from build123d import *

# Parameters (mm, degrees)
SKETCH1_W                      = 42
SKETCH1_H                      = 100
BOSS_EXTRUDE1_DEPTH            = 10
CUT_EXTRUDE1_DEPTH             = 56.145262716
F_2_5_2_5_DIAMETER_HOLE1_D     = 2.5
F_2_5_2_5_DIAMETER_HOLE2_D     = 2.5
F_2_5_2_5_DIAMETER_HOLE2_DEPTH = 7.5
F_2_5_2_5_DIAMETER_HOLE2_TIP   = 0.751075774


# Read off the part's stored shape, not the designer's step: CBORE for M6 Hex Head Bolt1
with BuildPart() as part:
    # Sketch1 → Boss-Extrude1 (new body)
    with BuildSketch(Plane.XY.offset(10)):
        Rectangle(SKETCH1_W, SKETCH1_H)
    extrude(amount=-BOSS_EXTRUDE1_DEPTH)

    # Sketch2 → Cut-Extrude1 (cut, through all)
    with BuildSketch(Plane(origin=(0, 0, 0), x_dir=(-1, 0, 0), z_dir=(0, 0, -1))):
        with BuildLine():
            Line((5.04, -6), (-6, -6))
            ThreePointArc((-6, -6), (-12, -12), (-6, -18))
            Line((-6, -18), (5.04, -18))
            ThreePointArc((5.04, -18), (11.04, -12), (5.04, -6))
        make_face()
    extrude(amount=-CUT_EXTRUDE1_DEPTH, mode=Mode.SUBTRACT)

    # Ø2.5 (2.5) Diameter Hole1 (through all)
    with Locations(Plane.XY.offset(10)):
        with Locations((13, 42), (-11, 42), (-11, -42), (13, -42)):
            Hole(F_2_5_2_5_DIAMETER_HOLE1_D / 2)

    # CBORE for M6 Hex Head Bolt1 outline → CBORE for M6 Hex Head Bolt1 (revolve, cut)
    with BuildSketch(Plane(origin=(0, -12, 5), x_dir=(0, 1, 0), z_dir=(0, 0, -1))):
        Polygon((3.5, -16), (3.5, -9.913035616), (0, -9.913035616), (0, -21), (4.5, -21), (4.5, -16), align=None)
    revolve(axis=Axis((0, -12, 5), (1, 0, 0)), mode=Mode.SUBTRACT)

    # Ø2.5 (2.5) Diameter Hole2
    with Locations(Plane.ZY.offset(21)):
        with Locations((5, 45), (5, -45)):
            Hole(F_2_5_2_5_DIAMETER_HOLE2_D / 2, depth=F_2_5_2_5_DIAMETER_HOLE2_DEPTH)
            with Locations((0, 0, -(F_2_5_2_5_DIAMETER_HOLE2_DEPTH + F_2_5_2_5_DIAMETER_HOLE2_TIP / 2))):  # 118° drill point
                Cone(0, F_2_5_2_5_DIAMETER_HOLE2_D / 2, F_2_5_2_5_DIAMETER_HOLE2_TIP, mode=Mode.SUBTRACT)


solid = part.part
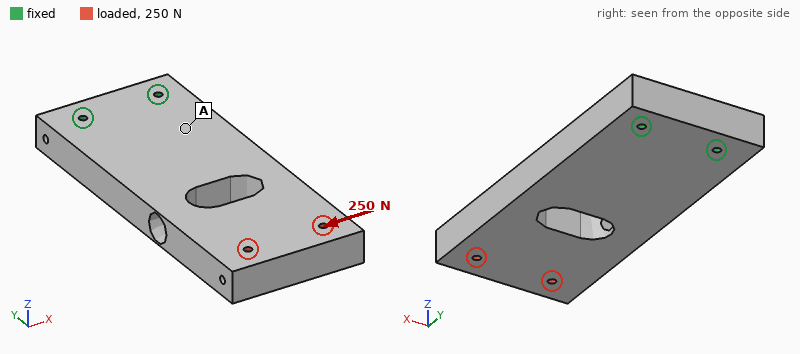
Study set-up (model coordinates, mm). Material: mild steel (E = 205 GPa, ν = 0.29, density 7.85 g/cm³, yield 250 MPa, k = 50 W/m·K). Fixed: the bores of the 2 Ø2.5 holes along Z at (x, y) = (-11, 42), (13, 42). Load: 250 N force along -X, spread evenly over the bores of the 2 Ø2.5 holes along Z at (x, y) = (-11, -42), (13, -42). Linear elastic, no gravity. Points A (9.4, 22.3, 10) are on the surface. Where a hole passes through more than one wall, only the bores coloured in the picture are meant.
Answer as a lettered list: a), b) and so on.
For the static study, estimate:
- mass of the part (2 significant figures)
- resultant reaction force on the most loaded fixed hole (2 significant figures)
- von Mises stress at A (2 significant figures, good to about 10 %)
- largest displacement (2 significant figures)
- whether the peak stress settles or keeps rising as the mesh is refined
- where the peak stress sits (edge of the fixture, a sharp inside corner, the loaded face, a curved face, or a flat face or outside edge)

a) 300 g
b) 850 N
c) 2.9 MPa
d) 8.2 µm
e) keeps rising
f) edge of the fixture
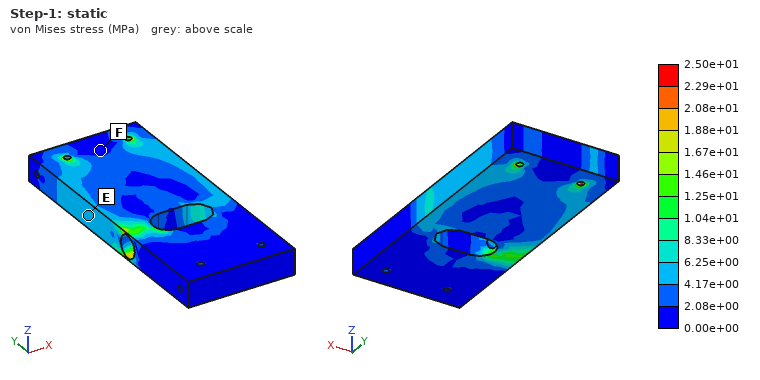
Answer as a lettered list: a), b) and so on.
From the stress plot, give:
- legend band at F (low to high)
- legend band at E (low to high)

a) 0.00e+00 to 2.08e+00 MPa
b) 4.17e+00 to 6.25e+00 MPa
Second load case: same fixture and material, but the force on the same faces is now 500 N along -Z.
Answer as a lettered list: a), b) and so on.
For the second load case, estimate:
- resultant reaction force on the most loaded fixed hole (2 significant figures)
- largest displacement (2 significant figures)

a) 260 N
b) 0.21 mm
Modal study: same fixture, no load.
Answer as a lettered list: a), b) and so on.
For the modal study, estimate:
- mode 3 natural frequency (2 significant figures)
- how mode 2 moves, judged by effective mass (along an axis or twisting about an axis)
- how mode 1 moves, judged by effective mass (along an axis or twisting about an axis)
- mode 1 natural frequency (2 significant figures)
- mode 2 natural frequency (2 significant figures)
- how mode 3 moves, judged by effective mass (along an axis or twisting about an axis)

a) 3700 Hz
b) along X
c) along Z
d) 890 Hz
e) 3000 Hz
f) twisting about Y
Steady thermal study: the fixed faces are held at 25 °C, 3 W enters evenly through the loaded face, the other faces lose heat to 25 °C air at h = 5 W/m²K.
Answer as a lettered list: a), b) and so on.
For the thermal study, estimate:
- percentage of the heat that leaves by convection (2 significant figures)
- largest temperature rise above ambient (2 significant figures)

a) 15 %
b) 17 K
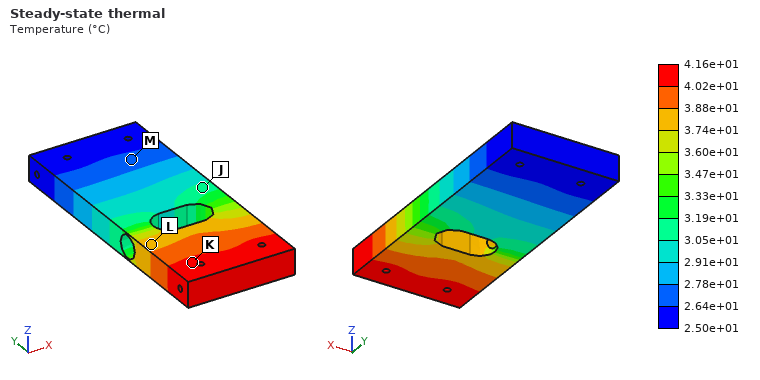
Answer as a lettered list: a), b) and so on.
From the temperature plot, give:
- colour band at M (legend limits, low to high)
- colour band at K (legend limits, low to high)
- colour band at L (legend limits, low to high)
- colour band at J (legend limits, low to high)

a) 2.64e+01 to 2.78e+01 °C
b) 4.02e+01 to 4.16e+01 °C
c) 3.74e+01 to 3.88e+01 °C
d) 3.05e+01 to 3.19e+01 °C
